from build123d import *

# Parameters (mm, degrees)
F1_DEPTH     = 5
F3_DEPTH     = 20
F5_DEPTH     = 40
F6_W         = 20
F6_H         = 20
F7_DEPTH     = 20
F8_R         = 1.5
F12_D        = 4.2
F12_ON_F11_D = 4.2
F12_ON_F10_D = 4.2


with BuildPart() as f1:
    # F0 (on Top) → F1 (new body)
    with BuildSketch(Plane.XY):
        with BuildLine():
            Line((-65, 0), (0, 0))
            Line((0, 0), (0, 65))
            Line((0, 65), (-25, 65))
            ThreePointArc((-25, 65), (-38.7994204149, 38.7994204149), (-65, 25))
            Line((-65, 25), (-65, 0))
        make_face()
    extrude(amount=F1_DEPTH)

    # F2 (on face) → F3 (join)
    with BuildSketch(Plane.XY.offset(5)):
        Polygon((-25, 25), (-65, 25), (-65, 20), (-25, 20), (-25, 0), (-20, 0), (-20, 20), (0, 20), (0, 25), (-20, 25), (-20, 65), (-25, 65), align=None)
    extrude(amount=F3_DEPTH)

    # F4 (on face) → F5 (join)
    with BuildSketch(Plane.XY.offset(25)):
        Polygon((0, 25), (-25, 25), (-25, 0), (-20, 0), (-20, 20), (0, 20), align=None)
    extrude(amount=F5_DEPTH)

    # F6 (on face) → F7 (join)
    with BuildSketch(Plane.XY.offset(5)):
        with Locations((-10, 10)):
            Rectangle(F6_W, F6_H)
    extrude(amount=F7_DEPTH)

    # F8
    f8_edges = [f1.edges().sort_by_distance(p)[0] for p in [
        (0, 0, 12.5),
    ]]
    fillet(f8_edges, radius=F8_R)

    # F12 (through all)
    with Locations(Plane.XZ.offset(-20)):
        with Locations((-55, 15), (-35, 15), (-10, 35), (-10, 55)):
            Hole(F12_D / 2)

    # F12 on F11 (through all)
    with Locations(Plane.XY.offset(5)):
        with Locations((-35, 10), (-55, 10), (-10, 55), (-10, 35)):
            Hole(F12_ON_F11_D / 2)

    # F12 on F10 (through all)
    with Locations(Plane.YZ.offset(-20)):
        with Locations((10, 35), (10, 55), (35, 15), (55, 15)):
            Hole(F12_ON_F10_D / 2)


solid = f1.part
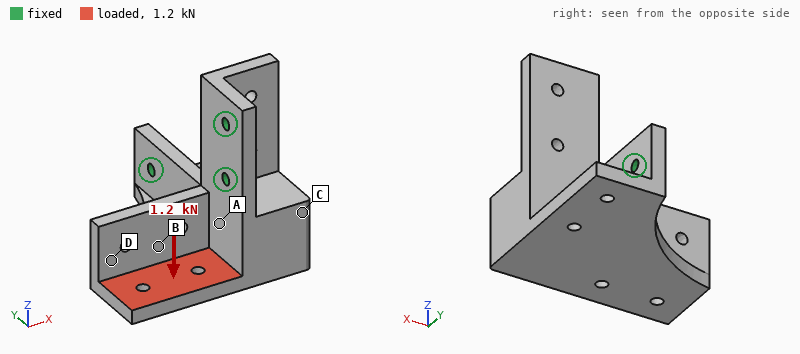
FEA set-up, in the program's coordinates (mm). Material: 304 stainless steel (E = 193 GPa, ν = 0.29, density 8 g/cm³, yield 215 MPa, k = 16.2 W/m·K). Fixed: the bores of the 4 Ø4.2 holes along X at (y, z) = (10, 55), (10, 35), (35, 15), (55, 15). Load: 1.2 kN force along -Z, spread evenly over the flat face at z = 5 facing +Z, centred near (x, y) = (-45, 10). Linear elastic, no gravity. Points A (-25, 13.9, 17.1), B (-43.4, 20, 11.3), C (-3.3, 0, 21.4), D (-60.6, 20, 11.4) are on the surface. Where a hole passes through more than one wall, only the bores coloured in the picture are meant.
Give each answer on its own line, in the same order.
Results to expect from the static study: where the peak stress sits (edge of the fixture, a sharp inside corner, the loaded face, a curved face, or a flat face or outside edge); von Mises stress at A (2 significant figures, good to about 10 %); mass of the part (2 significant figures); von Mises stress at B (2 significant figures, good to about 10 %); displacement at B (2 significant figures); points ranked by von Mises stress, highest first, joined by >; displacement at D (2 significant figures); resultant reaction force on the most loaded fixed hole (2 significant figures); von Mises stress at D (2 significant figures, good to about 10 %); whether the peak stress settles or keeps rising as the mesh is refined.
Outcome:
edge of the fixture
14 MPa
350 g
33 MPa
20 µm
B > D > A > C
35 µm
830 N
25 MPa
keeps rising
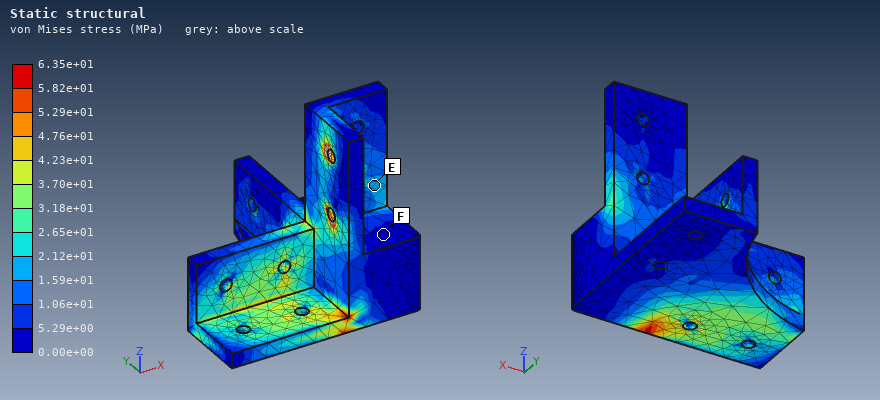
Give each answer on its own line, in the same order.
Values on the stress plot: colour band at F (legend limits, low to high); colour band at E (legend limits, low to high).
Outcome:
0.00e+00 to 5.29e+00 MPa
1.59e+01 to 2.12e+01 MPa
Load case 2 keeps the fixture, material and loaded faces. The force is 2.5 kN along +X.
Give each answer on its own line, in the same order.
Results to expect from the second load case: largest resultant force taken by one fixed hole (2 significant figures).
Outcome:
2.3 kN
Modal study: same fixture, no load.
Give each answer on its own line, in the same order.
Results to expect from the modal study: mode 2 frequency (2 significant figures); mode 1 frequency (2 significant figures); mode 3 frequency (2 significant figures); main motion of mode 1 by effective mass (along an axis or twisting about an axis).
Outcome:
5000 Hz
2600 Hz
5500 Hz
along X
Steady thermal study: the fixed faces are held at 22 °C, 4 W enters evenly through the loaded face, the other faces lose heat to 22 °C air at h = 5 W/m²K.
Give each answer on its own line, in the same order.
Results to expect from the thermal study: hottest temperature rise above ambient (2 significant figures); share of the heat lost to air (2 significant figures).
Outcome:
36 K
18 %
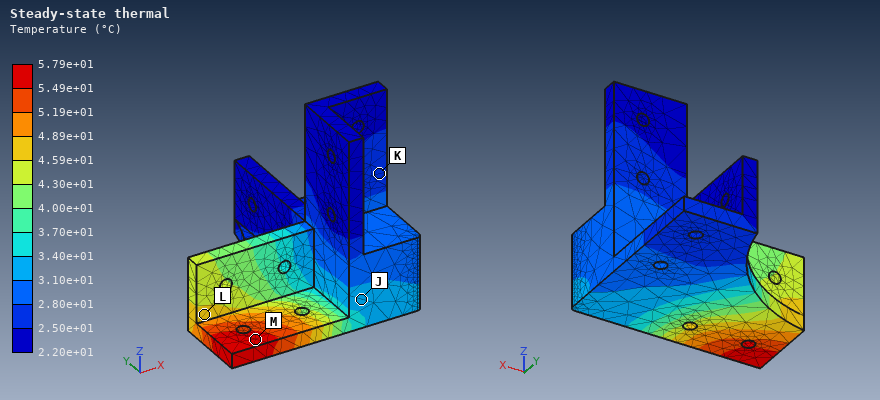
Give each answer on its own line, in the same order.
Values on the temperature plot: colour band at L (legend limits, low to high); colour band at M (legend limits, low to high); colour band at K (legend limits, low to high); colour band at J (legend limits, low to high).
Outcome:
4.59e+01 to 4.89e+01 °C
5.49e+01 to 5.79e+01 °C
2.50e+01 to 2.80e+01 °C
3.10e+01 to 3.40e+01 °C
